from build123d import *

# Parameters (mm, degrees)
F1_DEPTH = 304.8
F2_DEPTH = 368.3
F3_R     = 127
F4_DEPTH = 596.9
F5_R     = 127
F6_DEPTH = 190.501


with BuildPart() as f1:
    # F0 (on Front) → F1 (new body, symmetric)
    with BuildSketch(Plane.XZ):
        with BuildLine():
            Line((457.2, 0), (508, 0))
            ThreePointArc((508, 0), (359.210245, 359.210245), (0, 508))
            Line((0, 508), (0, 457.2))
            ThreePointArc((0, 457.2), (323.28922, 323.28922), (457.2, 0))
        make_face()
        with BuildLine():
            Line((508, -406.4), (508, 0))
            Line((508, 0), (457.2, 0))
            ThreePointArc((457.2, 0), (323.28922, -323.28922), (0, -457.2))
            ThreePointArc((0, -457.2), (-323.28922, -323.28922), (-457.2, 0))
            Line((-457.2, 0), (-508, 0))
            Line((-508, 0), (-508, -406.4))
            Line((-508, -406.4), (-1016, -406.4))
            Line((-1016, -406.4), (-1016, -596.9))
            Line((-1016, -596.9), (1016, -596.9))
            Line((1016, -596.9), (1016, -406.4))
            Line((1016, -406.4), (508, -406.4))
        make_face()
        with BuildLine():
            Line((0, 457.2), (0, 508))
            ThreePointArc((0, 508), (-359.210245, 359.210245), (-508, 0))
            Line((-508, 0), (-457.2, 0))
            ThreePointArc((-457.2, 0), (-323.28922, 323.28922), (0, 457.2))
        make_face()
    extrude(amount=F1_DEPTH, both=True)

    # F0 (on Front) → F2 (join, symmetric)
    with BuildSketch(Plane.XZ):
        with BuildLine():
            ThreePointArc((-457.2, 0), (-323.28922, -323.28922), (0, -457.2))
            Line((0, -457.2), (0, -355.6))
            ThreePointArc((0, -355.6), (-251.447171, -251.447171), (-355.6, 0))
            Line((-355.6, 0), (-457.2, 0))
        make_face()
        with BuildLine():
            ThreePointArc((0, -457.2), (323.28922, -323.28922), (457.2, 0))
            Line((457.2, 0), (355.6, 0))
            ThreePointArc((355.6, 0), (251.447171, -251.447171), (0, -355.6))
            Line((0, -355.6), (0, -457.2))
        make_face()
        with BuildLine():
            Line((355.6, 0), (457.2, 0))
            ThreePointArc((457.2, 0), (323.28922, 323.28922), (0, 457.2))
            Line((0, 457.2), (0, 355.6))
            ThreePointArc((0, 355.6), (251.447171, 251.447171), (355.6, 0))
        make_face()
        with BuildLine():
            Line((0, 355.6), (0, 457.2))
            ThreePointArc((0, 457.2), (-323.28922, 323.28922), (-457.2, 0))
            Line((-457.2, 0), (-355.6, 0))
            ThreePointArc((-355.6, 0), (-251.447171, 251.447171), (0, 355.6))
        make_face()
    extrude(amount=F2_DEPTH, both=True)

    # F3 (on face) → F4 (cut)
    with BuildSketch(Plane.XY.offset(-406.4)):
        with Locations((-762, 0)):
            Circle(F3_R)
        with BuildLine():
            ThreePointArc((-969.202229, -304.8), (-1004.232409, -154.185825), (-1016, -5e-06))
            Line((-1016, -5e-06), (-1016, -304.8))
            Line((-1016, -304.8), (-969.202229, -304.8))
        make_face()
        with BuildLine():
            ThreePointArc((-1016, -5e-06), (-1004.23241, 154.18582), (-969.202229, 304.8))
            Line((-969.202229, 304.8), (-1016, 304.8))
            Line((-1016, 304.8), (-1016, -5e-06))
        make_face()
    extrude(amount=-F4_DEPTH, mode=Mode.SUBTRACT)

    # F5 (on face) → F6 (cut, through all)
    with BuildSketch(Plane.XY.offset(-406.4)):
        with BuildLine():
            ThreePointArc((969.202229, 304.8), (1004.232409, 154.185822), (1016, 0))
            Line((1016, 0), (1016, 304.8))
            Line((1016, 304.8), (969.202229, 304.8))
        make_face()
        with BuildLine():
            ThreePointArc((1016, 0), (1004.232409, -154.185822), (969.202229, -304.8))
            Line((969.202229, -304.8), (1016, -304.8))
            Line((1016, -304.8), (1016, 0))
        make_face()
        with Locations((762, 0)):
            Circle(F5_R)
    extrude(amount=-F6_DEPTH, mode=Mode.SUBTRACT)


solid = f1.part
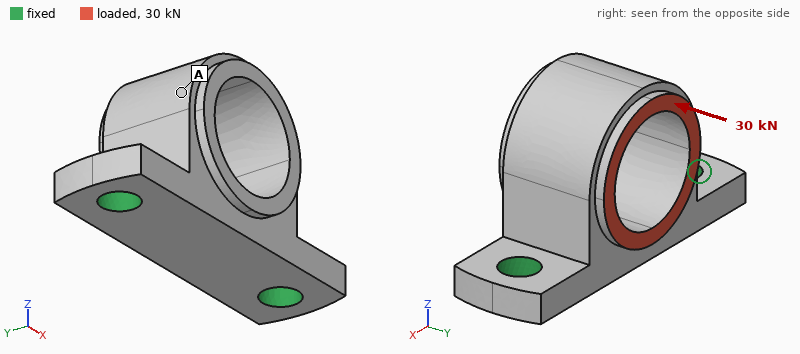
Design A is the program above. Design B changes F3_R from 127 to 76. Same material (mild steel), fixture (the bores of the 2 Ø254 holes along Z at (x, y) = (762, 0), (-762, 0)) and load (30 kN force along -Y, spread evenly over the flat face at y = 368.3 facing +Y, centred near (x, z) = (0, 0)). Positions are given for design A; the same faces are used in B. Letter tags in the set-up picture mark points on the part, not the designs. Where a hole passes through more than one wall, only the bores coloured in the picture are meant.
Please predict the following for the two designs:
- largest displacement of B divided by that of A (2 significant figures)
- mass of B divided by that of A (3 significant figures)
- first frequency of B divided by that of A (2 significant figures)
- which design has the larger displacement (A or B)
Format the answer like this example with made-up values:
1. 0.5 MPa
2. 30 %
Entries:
1. 1.2
2. 1.01
3. 0.93
4. B
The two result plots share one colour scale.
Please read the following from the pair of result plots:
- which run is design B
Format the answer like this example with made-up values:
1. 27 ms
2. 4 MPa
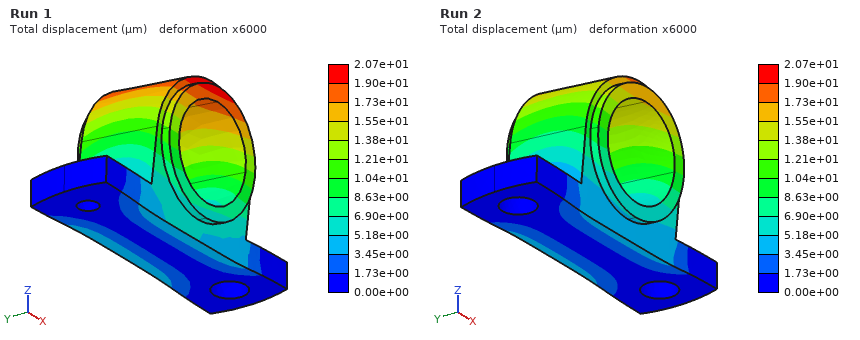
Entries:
1. Run 1
